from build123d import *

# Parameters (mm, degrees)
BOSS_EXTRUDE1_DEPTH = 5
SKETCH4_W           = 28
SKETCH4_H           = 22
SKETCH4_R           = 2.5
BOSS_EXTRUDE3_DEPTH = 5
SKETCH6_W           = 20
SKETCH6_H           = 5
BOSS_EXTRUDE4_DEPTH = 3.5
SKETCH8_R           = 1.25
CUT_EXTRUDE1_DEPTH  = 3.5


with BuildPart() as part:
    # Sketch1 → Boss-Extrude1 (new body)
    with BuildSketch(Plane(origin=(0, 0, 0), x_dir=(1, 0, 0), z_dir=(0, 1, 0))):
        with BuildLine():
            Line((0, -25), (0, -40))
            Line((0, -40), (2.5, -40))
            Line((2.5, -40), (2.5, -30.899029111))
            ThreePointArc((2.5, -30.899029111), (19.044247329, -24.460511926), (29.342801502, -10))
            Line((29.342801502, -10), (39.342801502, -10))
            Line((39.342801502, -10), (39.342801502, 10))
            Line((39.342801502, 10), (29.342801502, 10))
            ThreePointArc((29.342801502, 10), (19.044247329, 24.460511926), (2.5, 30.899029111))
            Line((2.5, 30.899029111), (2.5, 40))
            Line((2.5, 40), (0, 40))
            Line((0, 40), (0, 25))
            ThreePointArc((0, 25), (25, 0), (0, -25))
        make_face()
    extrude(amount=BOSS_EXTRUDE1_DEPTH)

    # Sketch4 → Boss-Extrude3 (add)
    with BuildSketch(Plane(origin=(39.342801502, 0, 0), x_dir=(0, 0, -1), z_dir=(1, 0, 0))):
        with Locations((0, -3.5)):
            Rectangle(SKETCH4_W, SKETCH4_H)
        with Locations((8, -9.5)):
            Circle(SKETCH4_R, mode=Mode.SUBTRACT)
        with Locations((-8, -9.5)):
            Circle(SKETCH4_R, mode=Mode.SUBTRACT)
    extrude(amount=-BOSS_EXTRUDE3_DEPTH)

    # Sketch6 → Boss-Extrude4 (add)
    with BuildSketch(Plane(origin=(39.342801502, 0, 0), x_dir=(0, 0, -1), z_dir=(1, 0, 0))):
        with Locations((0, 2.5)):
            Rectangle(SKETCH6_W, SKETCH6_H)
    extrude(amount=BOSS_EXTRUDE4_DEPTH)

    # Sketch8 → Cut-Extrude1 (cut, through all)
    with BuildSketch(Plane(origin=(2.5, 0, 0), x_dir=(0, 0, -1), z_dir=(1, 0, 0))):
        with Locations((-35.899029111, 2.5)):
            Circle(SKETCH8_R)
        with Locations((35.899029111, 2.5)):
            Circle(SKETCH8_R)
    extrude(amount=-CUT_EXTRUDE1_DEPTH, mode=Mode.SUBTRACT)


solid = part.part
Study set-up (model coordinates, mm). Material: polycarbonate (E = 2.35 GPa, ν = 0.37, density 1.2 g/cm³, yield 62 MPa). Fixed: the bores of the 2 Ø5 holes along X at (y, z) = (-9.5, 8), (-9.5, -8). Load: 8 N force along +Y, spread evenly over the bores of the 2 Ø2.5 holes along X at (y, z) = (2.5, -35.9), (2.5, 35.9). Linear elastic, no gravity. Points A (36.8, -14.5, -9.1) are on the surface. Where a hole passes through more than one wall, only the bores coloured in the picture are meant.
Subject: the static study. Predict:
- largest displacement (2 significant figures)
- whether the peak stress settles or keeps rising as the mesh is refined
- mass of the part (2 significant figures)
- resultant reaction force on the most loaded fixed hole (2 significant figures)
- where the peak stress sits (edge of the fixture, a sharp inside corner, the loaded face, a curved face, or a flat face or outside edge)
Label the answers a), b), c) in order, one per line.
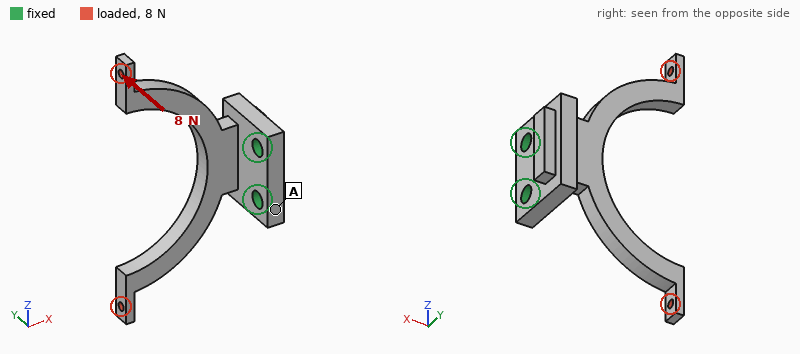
a) 1.0 mm
b) keeps rising
c) 7.8 g
d) 4.0 N
e) a sharp inside corner
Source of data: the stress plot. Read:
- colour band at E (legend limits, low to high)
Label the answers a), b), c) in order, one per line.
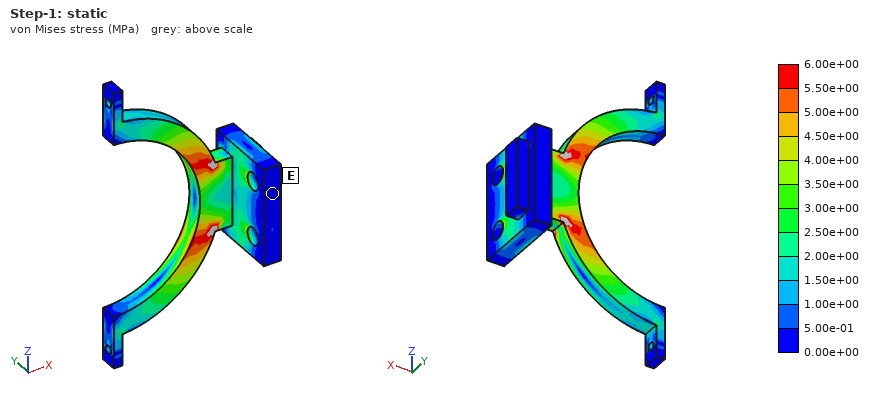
a) 0.00e+00 to 5.00e-01 MPa
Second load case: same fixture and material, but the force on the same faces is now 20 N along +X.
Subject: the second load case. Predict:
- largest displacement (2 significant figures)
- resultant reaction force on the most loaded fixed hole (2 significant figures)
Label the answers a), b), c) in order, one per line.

a) 0.97 mm
b) 10 N
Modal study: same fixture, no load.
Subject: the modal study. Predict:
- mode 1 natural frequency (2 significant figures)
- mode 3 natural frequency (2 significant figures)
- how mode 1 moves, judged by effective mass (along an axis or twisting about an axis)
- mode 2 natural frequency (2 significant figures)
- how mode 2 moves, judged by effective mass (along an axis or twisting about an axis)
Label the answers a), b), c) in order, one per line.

a) 510 Hz
b) 700 Hz
c) along Y
d) 550 Hz
e) twisting about X
